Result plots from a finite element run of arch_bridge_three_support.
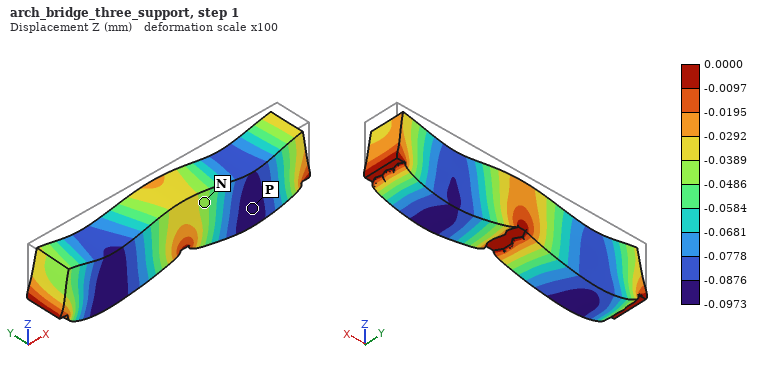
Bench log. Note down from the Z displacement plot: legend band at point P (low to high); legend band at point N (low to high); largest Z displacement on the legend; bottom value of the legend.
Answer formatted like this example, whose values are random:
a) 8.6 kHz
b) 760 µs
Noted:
a) -0.0973 to -0.0876 mm
b) -0.0486 to -0.0389 mm
c) 0.0000 mm
d) -0.0973 mm
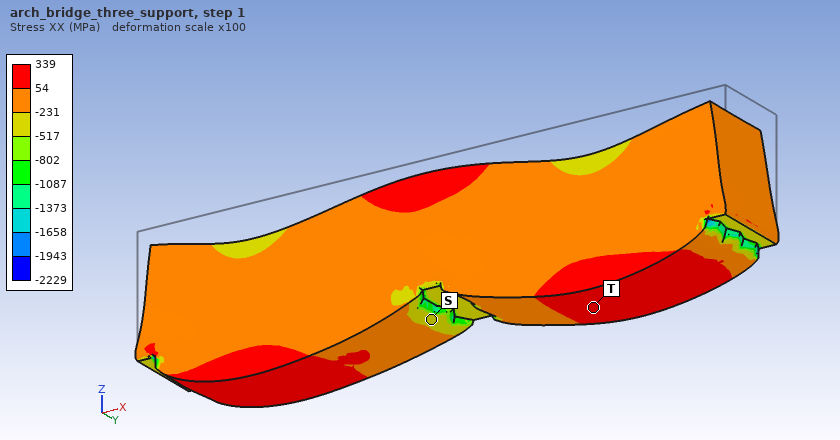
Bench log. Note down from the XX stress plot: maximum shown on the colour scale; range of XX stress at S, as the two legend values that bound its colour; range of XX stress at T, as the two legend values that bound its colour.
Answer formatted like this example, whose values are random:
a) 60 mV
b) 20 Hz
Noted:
a) 339 MPa
b) -517 to -231 MPa
c) 54 to 339 MPa
